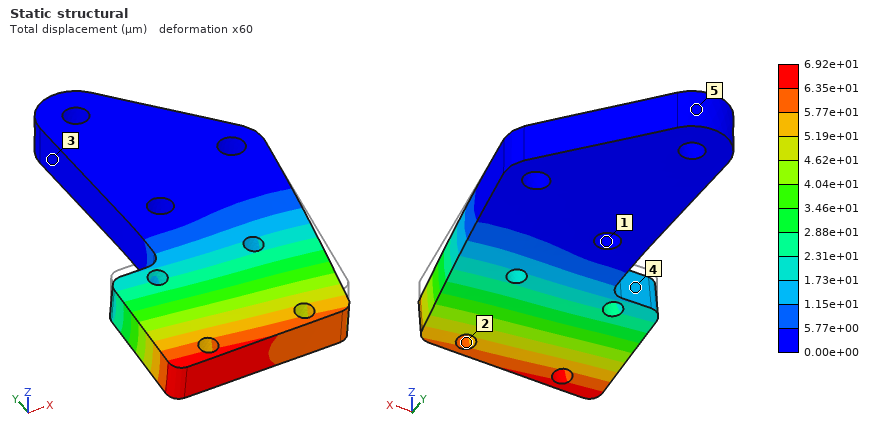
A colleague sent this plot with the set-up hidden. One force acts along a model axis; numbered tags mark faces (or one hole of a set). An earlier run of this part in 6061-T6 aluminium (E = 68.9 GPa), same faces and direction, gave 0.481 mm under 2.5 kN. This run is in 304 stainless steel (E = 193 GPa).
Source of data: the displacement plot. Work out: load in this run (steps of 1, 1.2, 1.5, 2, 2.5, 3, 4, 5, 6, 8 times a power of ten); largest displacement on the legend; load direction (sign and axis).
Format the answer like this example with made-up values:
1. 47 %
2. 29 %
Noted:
1. 1 kN
2. 6.92e+01 µm
3. -Z
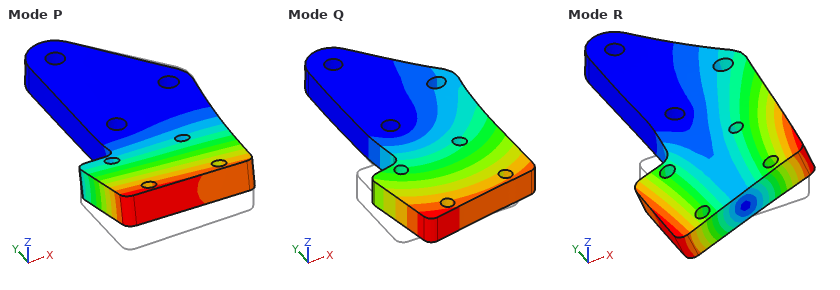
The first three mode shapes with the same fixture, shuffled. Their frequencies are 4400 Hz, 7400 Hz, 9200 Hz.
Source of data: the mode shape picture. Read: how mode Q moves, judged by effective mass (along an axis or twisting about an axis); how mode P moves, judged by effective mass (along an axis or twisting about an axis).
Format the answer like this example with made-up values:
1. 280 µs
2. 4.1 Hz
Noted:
1. along X
2. along Z
